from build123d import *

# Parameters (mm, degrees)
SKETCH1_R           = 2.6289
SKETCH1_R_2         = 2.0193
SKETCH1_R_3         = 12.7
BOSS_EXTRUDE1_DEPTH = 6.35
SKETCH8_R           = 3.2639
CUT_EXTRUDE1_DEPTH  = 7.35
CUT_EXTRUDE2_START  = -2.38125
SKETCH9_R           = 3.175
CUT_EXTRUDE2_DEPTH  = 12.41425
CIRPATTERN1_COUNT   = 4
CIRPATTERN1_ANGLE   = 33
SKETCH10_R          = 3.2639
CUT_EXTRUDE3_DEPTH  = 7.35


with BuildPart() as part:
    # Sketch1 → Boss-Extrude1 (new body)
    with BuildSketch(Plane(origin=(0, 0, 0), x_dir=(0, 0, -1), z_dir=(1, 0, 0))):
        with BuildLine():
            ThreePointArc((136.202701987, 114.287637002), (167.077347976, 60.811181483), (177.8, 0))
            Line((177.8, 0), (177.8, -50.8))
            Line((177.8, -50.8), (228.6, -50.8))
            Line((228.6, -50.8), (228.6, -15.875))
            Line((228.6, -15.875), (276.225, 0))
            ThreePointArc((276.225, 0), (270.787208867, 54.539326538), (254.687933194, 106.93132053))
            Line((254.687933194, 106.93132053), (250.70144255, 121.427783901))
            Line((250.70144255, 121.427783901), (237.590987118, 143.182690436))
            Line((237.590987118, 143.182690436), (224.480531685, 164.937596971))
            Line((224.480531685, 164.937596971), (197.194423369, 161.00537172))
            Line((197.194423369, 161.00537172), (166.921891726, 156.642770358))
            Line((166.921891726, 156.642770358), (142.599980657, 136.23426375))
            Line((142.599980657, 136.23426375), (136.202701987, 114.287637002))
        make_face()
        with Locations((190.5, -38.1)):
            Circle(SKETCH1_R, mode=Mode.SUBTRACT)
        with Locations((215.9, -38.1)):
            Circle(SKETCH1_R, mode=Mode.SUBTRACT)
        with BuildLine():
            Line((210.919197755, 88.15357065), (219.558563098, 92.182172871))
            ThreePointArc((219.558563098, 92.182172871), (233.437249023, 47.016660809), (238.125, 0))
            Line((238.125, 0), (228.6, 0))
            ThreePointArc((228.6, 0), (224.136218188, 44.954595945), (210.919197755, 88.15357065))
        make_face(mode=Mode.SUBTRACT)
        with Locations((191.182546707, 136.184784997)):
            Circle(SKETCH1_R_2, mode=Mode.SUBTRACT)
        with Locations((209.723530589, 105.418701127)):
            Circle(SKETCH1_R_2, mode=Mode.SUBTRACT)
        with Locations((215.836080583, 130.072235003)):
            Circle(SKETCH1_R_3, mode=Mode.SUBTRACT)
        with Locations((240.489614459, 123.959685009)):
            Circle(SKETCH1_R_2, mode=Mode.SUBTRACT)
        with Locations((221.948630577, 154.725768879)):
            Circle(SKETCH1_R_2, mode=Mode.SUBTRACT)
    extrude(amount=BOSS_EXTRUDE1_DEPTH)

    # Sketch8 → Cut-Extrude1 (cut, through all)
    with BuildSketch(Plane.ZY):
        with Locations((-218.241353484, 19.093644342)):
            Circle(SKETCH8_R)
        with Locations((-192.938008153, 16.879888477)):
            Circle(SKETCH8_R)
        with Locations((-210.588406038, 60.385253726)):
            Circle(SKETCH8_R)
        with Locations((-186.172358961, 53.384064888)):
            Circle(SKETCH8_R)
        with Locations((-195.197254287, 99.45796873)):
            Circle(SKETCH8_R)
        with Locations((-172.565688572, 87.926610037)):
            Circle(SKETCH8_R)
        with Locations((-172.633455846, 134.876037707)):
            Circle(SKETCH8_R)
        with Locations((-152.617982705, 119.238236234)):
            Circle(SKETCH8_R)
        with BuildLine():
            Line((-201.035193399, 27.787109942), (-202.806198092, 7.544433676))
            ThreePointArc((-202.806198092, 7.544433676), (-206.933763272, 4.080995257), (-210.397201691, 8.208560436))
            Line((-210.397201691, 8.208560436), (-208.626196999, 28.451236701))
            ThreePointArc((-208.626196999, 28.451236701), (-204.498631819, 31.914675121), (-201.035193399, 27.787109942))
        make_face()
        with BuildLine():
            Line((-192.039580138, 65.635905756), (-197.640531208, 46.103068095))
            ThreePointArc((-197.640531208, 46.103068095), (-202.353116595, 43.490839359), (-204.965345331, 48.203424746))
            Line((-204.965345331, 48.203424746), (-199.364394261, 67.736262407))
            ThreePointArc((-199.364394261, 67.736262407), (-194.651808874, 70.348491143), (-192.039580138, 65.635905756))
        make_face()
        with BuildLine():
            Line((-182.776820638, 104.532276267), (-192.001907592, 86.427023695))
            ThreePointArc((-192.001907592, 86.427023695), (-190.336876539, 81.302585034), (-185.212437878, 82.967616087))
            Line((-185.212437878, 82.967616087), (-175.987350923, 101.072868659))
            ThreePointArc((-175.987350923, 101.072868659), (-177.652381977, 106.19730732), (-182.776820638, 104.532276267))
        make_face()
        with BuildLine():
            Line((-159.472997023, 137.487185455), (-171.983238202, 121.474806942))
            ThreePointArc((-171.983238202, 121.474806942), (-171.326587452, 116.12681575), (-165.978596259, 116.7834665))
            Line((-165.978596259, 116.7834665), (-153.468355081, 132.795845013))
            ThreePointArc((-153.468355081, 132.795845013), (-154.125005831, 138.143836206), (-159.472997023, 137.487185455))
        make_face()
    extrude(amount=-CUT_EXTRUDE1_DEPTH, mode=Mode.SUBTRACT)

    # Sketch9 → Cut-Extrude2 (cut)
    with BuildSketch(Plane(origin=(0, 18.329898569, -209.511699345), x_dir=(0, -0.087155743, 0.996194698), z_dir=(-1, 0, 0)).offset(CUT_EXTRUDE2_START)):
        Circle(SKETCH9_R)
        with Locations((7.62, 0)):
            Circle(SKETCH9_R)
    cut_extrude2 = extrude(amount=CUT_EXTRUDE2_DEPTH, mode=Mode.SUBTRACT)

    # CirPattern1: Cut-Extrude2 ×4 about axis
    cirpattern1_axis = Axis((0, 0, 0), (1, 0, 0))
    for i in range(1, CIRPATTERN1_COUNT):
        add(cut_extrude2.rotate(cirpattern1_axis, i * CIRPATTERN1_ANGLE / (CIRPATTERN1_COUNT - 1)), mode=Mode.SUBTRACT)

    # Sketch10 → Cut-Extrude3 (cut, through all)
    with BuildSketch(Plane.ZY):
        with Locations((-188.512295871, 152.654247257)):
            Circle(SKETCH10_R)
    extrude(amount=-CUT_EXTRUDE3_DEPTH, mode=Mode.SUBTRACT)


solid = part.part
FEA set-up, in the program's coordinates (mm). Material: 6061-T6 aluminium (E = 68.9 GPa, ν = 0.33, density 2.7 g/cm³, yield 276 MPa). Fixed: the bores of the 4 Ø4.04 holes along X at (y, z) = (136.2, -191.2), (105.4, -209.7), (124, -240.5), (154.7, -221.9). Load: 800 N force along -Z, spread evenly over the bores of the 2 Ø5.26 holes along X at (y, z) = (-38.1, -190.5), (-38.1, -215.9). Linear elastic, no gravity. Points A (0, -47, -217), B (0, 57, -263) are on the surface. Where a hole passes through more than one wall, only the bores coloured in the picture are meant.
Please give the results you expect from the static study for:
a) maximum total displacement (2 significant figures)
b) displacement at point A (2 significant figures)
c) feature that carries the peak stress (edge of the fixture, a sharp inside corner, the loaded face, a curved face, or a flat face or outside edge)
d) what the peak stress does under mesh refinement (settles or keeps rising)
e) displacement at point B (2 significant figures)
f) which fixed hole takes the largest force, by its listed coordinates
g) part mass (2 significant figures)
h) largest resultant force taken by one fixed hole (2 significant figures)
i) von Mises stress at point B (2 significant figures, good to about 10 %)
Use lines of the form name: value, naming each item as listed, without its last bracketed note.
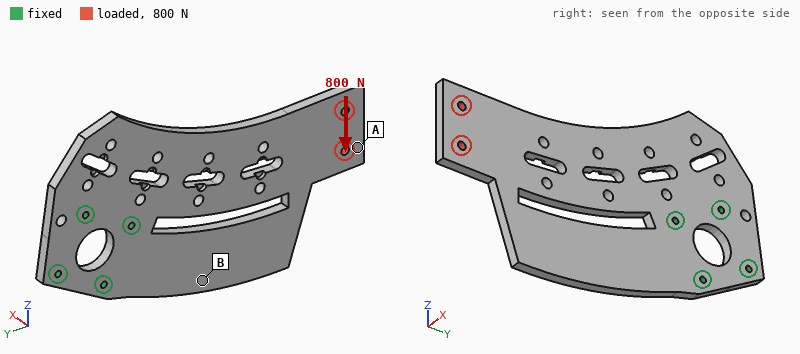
maximum total displacement: 0.11 mm
displacement at point A: 0.11 mm
feature that carries the peak stress: edge of the fixture
what the peak stress does under mesh refinement: keeps rising
displacement at point B: 0.038 mm
which fixed hole takes the largest force, by its listed coordinates: (105.4, -209.7)
part mass: 280 g
largest resultant force taken by one fixed hole: 1.9 kN
von Mises stress at point B: 6.5 MPa
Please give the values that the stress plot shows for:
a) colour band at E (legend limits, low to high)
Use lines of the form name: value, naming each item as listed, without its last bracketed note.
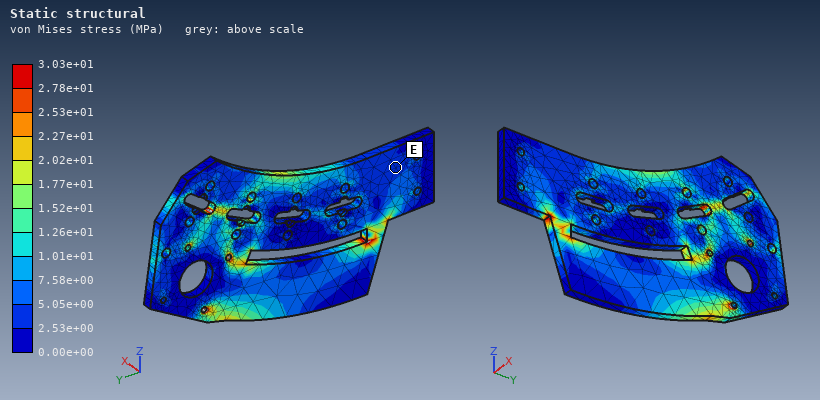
colour band at E: 2.53e+00 to 5.05e+00 MPa
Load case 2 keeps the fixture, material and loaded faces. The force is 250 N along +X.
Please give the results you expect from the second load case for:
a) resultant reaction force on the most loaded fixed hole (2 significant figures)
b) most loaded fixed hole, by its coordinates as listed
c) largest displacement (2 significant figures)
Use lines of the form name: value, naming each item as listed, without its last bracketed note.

resultant reaction force on the most loaded fixed hole: 940 N
most loaded fixed hole, by its coordinates as listed: (105.4, -209.7)
largest displacement: 3.0 mm
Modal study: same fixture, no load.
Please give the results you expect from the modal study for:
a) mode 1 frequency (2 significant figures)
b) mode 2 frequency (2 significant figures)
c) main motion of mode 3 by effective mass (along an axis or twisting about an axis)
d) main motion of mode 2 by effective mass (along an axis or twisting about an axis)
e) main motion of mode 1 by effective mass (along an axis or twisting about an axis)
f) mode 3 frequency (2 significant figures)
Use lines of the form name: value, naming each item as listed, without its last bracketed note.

mode 1 frequency: 220 Hz
mode 2 frequency: 640 Hz
main motion of mode 3 by effective mass: along X
main motion of mode 2 by effective mass: twisting about Y
main motion of mode 1 by effective mass: along X
mode 3 frequency: 1200 Hz
